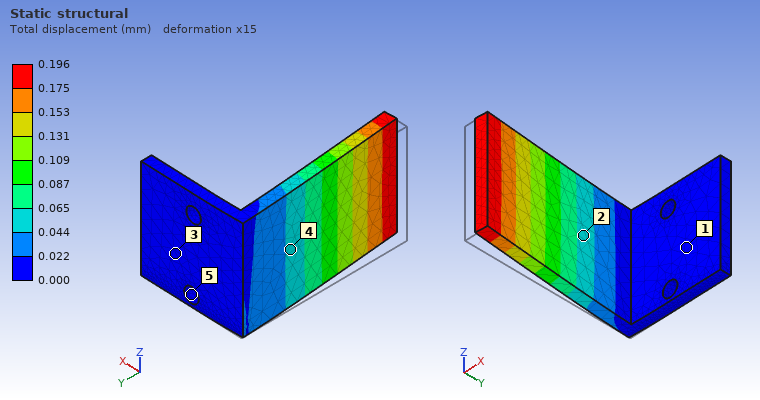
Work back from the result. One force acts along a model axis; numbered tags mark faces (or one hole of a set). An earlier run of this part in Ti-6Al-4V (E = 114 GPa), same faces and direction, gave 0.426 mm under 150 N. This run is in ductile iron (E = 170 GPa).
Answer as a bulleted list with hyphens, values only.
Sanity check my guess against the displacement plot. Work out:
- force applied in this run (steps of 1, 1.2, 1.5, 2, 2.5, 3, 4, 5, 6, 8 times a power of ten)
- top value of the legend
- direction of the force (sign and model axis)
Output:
- 100 N
- 0.196 mm
- +X
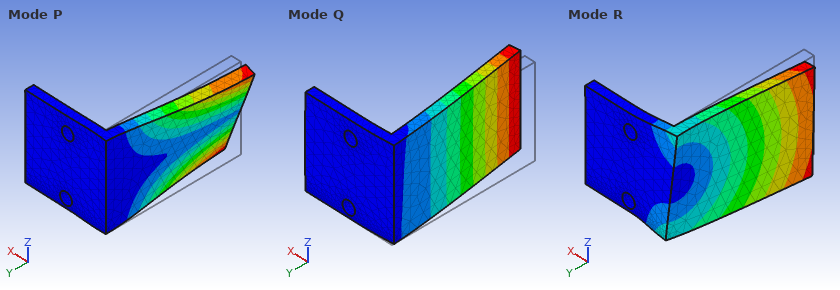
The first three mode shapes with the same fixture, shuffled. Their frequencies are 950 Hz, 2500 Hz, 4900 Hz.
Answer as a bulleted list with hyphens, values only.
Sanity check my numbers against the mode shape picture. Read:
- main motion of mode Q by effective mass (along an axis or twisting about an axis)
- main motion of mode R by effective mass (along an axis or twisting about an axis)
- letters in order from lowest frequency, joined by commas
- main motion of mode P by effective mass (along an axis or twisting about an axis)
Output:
- along X
- along Z
- Q, R, P
- twisting about Y
